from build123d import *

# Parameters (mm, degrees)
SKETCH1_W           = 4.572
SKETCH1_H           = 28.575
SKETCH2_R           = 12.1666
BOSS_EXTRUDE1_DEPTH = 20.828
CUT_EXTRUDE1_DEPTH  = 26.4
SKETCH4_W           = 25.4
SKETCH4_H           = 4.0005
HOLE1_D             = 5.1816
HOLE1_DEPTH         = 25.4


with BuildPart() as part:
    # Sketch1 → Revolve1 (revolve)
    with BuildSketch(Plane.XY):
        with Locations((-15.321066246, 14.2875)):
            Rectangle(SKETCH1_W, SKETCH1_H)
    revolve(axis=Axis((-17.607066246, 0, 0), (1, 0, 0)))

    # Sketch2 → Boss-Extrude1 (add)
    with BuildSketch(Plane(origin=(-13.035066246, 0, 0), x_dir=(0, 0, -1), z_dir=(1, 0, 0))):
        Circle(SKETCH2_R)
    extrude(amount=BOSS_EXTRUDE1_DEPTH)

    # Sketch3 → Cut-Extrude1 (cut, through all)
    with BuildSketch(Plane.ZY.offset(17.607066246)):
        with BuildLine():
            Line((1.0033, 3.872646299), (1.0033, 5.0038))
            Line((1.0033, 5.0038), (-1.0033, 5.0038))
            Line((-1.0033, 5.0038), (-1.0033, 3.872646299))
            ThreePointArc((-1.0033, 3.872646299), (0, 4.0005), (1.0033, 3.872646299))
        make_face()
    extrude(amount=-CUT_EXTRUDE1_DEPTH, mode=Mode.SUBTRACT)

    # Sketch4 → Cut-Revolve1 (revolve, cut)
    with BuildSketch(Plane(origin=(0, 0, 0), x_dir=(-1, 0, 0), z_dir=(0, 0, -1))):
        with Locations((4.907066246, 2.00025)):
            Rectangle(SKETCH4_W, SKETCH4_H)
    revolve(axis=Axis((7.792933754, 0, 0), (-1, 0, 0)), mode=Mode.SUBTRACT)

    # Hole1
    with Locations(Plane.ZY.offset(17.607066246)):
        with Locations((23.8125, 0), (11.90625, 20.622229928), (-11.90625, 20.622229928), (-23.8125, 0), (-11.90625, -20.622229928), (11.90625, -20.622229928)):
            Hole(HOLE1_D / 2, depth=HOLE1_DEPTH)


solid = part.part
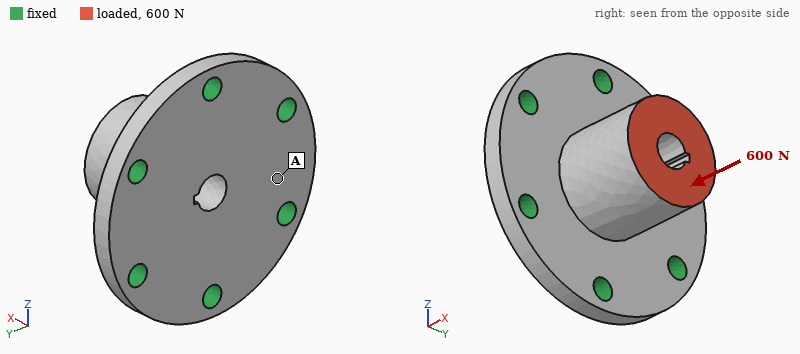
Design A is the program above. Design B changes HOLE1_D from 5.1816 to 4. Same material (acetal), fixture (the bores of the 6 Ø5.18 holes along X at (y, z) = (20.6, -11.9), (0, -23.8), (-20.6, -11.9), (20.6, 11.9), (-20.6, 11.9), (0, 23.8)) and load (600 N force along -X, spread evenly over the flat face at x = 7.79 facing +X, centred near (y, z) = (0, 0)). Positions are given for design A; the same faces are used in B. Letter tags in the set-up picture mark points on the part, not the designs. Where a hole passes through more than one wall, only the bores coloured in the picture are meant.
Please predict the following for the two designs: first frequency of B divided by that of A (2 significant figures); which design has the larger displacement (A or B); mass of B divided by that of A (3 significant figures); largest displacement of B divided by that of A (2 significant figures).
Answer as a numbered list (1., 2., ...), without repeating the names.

1. 0.96
2. B
3. 1.01
4. 1.1
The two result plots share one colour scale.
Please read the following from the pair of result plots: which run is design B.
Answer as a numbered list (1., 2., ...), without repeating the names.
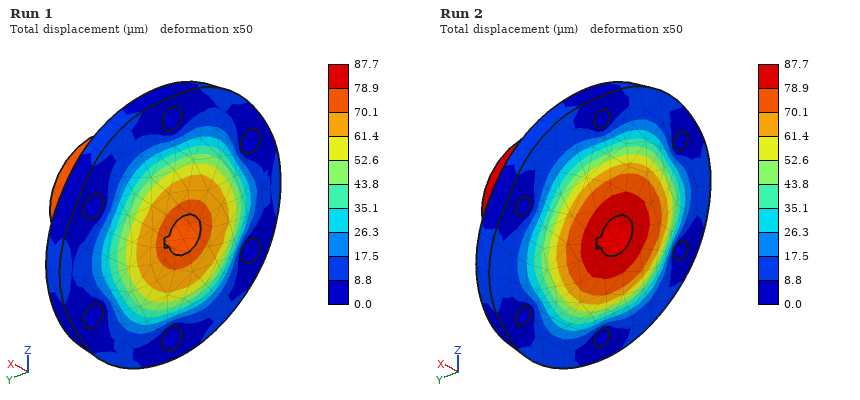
1. Run 2
